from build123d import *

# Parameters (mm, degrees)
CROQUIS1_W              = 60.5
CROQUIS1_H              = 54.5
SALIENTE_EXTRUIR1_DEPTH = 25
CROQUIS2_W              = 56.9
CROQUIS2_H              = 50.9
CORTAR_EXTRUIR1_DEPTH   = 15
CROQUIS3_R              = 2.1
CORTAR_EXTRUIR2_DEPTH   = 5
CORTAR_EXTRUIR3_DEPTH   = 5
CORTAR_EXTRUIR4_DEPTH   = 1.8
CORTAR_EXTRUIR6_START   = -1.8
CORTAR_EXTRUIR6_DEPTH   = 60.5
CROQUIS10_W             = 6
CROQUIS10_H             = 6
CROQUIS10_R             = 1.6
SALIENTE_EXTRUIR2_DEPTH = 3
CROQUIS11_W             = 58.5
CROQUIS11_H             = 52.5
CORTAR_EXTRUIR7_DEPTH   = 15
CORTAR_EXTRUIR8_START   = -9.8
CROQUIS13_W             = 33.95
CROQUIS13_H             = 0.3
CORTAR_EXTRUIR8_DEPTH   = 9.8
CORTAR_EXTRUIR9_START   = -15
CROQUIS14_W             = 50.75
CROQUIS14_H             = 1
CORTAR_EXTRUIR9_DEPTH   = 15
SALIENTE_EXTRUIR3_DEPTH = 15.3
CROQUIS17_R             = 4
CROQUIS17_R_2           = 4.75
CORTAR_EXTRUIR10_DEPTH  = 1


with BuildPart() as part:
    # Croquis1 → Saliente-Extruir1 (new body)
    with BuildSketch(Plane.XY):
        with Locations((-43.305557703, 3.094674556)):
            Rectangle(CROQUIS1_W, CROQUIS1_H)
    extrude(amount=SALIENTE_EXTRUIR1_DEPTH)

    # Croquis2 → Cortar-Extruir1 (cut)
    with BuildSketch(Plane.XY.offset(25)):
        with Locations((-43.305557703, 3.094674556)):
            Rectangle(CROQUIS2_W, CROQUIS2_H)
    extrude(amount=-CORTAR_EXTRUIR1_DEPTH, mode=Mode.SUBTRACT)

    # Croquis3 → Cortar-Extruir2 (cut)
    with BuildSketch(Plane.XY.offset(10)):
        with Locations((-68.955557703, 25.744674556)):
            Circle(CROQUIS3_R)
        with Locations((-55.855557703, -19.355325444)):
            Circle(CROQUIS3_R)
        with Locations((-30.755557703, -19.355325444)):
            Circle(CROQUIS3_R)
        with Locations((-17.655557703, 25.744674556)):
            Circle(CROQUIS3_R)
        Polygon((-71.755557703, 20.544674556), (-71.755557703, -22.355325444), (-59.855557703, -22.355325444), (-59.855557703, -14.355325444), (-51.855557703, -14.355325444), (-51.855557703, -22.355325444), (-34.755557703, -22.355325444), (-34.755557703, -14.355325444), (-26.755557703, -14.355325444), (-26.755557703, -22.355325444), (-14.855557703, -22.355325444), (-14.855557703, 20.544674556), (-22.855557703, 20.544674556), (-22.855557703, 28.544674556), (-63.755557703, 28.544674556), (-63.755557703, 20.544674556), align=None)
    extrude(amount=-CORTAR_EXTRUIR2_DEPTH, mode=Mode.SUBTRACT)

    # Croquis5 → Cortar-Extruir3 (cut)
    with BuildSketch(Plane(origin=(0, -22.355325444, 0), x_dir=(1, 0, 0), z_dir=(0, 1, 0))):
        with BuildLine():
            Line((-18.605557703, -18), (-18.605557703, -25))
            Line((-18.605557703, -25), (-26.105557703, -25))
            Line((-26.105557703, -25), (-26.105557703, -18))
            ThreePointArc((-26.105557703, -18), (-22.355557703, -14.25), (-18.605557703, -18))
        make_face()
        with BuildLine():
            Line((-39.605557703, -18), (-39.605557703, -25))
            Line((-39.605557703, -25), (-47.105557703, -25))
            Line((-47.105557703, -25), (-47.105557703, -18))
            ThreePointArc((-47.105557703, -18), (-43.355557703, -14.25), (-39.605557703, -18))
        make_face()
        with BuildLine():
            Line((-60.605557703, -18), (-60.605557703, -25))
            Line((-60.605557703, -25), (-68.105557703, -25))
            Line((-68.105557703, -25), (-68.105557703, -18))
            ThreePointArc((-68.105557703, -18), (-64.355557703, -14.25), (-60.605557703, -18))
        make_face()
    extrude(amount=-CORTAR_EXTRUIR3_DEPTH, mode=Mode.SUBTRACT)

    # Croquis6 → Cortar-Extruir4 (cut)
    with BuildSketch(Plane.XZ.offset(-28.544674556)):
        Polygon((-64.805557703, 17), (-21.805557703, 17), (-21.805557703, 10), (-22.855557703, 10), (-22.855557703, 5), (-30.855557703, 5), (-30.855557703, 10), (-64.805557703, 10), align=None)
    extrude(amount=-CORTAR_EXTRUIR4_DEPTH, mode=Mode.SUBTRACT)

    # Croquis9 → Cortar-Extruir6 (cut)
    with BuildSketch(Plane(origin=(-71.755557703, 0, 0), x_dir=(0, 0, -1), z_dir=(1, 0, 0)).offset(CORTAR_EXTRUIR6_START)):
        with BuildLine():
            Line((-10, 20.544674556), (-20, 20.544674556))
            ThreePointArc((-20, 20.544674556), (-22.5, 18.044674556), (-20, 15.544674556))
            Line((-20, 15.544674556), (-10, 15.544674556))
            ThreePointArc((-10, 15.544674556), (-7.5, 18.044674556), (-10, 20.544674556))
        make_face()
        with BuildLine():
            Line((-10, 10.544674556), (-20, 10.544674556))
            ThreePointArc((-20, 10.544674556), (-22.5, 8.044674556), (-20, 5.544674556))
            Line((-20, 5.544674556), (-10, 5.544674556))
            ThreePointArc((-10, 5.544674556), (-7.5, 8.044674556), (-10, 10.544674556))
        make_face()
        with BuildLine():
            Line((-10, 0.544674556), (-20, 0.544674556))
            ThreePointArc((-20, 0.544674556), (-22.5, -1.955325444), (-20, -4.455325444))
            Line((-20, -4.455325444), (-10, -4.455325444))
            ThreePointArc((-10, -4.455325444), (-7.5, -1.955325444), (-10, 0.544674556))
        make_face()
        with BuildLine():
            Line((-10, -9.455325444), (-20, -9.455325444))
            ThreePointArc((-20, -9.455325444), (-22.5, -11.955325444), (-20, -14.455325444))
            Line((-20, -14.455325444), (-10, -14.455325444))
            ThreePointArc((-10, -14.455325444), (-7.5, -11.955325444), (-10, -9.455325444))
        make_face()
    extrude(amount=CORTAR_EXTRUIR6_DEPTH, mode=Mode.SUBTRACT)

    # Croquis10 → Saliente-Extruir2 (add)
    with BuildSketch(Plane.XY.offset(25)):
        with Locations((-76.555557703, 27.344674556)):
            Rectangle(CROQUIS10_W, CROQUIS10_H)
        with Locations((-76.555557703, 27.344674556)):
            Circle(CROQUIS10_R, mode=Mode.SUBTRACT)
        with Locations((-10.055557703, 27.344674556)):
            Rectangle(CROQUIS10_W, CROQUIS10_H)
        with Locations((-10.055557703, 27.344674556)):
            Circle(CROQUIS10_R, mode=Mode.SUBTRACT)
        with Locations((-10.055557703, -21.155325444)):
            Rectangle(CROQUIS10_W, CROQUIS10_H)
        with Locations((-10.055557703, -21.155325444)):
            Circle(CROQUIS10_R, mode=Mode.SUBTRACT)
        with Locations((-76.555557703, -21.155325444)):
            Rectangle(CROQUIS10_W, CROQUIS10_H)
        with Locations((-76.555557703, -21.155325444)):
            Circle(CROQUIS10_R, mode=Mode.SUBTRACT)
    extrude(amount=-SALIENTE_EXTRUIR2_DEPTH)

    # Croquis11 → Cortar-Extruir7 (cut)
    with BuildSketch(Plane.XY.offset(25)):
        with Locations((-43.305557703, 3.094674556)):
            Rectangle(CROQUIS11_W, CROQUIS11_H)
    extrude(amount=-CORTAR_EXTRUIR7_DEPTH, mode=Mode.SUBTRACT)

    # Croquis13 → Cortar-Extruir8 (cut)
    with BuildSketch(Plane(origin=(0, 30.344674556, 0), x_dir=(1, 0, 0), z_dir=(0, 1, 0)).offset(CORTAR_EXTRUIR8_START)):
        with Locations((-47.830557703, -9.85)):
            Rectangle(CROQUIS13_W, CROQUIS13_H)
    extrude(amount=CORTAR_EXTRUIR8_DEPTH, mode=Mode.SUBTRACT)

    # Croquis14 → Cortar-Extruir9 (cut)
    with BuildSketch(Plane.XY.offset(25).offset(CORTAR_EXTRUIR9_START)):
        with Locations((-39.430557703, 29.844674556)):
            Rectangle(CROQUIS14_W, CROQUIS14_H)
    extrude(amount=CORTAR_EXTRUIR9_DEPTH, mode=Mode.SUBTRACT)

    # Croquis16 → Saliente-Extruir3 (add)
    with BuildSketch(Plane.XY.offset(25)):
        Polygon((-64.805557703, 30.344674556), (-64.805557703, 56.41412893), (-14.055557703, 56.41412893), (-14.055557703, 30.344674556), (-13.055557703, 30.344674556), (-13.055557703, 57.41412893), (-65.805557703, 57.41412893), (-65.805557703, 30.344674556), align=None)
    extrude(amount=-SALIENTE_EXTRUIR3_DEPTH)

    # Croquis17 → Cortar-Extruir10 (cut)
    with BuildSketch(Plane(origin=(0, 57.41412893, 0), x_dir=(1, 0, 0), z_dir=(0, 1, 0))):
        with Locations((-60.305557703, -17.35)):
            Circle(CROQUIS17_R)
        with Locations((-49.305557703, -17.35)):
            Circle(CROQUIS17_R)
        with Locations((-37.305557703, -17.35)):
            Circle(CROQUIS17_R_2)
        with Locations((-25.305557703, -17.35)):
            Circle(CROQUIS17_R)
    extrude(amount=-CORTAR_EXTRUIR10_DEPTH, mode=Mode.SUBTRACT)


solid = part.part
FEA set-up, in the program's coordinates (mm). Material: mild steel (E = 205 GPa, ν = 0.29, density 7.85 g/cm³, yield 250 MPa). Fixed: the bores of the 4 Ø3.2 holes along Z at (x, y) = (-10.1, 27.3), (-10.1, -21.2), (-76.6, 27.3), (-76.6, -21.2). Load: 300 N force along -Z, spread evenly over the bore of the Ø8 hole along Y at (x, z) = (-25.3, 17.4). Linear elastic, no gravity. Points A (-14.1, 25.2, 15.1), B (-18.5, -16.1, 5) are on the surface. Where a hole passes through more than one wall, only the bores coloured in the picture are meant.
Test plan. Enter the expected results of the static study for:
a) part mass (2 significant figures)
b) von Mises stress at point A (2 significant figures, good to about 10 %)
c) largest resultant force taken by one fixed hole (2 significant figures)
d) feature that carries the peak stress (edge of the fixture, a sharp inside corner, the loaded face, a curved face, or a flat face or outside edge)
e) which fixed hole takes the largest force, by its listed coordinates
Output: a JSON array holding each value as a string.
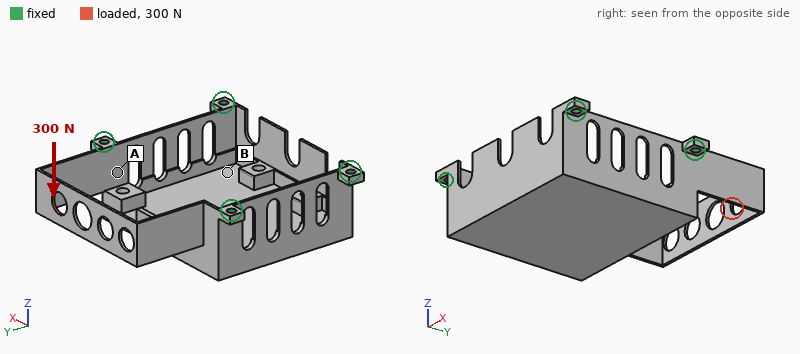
["180 g", "64 MPa", "380 N", "a flat face or outside edge", "(-10.1, 27.3)"]
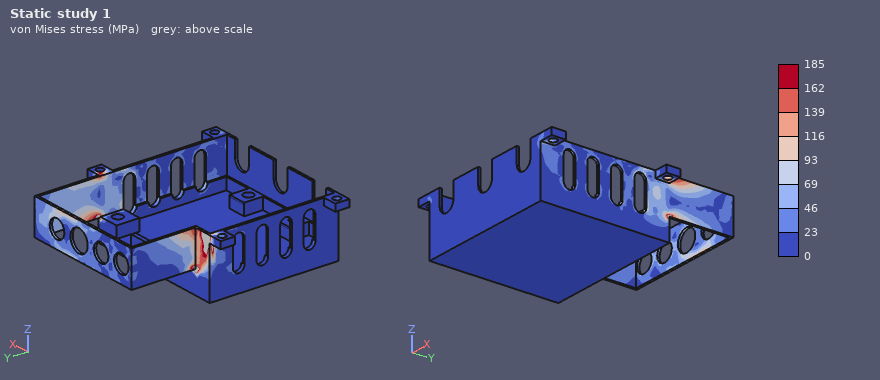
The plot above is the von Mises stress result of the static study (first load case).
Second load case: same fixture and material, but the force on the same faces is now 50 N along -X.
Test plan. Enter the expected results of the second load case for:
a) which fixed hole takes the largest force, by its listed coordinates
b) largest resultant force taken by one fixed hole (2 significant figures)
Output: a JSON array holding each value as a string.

["(-10.1, 27.3)", "30 N"]
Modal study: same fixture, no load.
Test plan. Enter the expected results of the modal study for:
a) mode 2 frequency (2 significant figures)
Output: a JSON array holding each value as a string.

["1500 Hz"]
